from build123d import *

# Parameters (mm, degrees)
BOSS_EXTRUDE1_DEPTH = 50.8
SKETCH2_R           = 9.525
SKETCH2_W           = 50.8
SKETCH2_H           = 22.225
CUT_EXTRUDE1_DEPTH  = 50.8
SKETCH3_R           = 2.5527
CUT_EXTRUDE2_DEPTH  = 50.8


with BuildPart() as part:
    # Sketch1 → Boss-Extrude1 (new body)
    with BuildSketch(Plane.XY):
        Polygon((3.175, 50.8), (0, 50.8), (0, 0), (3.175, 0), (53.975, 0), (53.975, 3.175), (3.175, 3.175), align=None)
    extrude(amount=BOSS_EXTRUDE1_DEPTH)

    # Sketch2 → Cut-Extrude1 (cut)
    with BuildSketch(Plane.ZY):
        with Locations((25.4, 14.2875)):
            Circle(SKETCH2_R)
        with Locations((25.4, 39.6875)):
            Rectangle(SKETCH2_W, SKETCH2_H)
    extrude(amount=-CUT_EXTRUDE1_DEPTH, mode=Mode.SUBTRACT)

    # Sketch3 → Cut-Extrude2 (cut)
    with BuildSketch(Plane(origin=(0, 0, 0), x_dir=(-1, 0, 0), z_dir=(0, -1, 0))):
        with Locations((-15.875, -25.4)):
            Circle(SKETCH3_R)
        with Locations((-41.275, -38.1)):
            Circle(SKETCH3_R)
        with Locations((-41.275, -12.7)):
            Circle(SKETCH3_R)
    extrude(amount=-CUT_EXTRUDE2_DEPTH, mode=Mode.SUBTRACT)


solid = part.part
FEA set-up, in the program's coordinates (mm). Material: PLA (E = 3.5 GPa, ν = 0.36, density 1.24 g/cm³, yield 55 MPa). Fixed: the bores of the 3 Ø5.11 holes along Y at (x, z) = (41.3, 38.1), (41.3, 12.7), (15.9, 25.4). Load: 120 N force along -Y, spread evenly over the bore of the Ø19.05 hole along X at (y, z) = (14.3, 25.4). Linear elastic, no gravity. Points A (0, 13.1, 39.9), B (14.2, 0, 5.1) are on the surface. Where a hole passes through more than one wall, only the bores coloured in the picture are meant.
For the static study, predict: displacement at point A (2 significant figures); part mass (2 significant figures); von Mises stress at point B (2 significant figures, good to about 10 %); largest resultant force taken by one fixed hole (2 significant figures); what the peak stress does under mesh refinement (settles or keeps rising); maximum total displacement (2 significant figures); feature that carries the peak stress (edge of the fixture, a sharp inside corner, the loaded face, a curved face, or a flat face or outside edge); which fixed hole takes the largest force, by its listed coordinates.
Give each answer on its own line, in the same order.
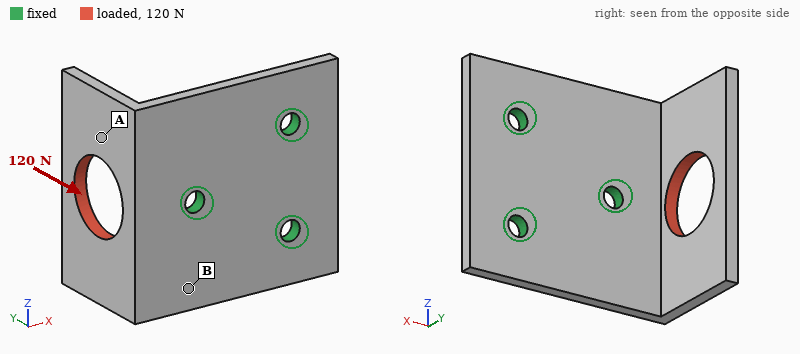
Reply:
0.51 mm
15 g
6.6 MPa
140 N
keeps rising
0.86 mm
edge of the fixture
(15.9, 25.4)
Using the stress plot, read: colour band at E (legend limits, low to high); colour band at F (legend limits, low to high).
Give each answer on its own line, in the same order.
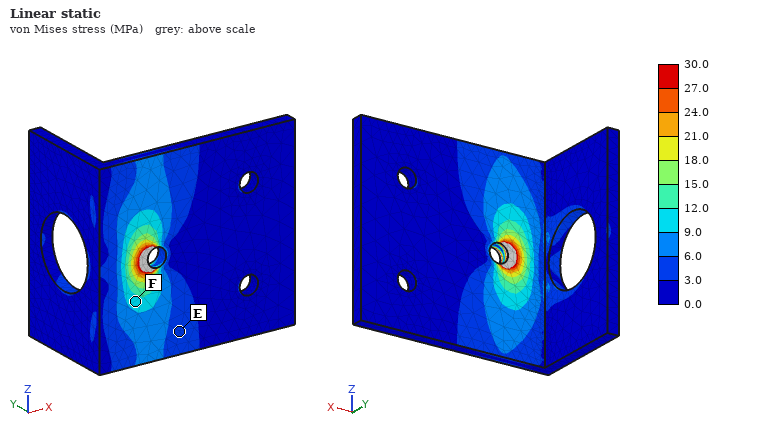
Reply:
3.0 to 6.0 MPa
9.0 to 12.0 MPa
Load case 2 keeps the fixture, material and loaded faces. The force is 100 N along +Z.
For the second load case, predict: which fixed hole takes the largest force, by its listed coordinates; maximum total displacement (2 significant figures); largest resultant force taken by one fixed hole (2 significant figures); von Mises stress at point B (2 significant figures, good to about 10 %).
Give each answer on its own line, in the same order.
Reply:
(15.9, 25.4)
0.95 mm
120 N
5.5 MPa
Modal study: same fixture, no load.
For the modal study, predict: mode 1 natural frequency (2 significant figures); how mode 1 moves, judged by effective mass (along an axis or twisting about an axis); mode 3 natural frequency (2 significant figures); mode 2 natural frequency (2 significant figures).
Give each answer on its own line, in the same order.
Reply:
650 Hz
along X
1400 Hz
700 Hz
